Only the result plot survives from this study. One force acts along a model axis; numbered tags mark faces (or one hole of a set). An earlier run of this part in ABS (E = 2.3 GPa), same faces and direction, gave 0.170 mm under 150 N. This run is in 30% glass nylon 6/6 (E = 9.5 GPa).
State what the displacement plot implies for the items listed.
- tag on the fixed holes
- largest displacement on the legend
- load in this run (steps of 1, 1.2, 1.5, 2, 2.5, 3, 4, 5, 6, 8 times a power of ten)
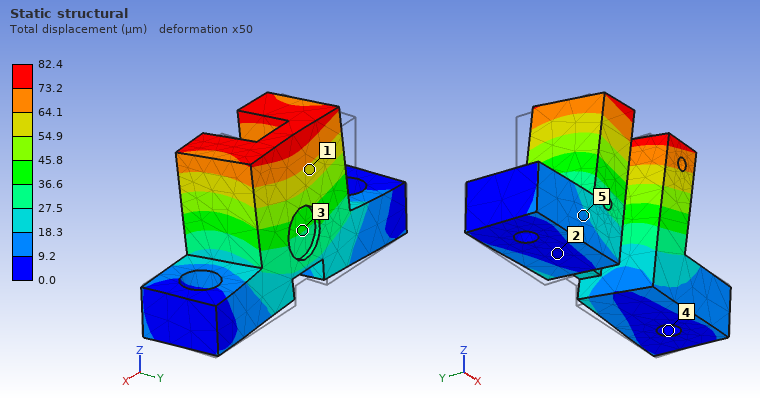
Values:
4
82.4 µm
300 N
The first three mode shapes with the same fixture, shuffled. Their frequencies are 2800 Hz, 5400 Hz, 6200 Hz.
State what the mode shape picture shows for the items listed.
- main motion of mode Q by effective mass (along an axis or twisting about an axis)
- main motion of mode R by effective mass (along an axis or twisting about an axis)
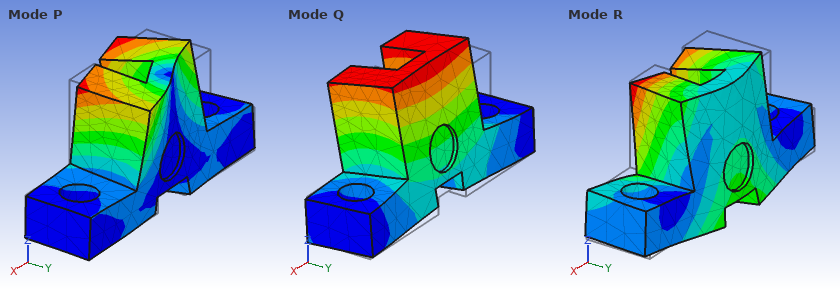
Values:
along Y
along Z
